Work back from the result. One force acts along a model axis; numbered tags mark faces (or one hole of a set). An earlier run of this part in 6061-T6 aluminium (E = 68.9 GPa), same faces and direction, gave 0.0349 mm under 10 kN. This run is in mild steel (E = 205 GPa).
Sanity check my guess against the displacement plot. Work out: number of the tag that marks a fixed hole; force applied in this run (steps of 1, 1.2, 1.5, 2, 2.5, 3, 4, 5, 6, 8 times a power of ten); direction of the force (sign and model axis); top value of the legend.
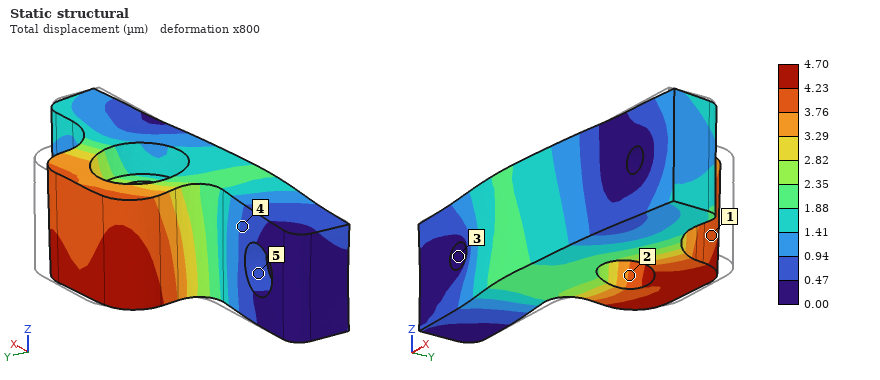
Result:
3
4 kN
-X
4.70 µm
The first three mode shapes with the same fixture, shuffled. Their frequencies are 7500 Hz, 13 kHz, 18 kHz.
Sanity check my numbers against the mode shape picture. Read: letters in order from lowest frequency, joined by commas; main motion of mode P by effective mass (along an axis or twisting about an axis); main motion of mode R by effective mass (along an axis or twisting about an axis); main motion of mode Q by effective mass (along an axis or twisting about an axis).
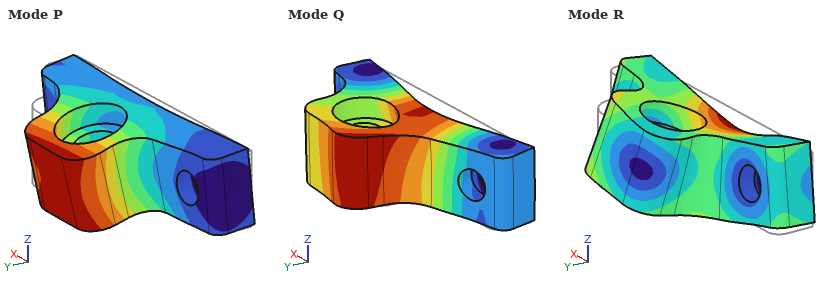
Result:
P, Q, R
along Z
along Z
along Y
